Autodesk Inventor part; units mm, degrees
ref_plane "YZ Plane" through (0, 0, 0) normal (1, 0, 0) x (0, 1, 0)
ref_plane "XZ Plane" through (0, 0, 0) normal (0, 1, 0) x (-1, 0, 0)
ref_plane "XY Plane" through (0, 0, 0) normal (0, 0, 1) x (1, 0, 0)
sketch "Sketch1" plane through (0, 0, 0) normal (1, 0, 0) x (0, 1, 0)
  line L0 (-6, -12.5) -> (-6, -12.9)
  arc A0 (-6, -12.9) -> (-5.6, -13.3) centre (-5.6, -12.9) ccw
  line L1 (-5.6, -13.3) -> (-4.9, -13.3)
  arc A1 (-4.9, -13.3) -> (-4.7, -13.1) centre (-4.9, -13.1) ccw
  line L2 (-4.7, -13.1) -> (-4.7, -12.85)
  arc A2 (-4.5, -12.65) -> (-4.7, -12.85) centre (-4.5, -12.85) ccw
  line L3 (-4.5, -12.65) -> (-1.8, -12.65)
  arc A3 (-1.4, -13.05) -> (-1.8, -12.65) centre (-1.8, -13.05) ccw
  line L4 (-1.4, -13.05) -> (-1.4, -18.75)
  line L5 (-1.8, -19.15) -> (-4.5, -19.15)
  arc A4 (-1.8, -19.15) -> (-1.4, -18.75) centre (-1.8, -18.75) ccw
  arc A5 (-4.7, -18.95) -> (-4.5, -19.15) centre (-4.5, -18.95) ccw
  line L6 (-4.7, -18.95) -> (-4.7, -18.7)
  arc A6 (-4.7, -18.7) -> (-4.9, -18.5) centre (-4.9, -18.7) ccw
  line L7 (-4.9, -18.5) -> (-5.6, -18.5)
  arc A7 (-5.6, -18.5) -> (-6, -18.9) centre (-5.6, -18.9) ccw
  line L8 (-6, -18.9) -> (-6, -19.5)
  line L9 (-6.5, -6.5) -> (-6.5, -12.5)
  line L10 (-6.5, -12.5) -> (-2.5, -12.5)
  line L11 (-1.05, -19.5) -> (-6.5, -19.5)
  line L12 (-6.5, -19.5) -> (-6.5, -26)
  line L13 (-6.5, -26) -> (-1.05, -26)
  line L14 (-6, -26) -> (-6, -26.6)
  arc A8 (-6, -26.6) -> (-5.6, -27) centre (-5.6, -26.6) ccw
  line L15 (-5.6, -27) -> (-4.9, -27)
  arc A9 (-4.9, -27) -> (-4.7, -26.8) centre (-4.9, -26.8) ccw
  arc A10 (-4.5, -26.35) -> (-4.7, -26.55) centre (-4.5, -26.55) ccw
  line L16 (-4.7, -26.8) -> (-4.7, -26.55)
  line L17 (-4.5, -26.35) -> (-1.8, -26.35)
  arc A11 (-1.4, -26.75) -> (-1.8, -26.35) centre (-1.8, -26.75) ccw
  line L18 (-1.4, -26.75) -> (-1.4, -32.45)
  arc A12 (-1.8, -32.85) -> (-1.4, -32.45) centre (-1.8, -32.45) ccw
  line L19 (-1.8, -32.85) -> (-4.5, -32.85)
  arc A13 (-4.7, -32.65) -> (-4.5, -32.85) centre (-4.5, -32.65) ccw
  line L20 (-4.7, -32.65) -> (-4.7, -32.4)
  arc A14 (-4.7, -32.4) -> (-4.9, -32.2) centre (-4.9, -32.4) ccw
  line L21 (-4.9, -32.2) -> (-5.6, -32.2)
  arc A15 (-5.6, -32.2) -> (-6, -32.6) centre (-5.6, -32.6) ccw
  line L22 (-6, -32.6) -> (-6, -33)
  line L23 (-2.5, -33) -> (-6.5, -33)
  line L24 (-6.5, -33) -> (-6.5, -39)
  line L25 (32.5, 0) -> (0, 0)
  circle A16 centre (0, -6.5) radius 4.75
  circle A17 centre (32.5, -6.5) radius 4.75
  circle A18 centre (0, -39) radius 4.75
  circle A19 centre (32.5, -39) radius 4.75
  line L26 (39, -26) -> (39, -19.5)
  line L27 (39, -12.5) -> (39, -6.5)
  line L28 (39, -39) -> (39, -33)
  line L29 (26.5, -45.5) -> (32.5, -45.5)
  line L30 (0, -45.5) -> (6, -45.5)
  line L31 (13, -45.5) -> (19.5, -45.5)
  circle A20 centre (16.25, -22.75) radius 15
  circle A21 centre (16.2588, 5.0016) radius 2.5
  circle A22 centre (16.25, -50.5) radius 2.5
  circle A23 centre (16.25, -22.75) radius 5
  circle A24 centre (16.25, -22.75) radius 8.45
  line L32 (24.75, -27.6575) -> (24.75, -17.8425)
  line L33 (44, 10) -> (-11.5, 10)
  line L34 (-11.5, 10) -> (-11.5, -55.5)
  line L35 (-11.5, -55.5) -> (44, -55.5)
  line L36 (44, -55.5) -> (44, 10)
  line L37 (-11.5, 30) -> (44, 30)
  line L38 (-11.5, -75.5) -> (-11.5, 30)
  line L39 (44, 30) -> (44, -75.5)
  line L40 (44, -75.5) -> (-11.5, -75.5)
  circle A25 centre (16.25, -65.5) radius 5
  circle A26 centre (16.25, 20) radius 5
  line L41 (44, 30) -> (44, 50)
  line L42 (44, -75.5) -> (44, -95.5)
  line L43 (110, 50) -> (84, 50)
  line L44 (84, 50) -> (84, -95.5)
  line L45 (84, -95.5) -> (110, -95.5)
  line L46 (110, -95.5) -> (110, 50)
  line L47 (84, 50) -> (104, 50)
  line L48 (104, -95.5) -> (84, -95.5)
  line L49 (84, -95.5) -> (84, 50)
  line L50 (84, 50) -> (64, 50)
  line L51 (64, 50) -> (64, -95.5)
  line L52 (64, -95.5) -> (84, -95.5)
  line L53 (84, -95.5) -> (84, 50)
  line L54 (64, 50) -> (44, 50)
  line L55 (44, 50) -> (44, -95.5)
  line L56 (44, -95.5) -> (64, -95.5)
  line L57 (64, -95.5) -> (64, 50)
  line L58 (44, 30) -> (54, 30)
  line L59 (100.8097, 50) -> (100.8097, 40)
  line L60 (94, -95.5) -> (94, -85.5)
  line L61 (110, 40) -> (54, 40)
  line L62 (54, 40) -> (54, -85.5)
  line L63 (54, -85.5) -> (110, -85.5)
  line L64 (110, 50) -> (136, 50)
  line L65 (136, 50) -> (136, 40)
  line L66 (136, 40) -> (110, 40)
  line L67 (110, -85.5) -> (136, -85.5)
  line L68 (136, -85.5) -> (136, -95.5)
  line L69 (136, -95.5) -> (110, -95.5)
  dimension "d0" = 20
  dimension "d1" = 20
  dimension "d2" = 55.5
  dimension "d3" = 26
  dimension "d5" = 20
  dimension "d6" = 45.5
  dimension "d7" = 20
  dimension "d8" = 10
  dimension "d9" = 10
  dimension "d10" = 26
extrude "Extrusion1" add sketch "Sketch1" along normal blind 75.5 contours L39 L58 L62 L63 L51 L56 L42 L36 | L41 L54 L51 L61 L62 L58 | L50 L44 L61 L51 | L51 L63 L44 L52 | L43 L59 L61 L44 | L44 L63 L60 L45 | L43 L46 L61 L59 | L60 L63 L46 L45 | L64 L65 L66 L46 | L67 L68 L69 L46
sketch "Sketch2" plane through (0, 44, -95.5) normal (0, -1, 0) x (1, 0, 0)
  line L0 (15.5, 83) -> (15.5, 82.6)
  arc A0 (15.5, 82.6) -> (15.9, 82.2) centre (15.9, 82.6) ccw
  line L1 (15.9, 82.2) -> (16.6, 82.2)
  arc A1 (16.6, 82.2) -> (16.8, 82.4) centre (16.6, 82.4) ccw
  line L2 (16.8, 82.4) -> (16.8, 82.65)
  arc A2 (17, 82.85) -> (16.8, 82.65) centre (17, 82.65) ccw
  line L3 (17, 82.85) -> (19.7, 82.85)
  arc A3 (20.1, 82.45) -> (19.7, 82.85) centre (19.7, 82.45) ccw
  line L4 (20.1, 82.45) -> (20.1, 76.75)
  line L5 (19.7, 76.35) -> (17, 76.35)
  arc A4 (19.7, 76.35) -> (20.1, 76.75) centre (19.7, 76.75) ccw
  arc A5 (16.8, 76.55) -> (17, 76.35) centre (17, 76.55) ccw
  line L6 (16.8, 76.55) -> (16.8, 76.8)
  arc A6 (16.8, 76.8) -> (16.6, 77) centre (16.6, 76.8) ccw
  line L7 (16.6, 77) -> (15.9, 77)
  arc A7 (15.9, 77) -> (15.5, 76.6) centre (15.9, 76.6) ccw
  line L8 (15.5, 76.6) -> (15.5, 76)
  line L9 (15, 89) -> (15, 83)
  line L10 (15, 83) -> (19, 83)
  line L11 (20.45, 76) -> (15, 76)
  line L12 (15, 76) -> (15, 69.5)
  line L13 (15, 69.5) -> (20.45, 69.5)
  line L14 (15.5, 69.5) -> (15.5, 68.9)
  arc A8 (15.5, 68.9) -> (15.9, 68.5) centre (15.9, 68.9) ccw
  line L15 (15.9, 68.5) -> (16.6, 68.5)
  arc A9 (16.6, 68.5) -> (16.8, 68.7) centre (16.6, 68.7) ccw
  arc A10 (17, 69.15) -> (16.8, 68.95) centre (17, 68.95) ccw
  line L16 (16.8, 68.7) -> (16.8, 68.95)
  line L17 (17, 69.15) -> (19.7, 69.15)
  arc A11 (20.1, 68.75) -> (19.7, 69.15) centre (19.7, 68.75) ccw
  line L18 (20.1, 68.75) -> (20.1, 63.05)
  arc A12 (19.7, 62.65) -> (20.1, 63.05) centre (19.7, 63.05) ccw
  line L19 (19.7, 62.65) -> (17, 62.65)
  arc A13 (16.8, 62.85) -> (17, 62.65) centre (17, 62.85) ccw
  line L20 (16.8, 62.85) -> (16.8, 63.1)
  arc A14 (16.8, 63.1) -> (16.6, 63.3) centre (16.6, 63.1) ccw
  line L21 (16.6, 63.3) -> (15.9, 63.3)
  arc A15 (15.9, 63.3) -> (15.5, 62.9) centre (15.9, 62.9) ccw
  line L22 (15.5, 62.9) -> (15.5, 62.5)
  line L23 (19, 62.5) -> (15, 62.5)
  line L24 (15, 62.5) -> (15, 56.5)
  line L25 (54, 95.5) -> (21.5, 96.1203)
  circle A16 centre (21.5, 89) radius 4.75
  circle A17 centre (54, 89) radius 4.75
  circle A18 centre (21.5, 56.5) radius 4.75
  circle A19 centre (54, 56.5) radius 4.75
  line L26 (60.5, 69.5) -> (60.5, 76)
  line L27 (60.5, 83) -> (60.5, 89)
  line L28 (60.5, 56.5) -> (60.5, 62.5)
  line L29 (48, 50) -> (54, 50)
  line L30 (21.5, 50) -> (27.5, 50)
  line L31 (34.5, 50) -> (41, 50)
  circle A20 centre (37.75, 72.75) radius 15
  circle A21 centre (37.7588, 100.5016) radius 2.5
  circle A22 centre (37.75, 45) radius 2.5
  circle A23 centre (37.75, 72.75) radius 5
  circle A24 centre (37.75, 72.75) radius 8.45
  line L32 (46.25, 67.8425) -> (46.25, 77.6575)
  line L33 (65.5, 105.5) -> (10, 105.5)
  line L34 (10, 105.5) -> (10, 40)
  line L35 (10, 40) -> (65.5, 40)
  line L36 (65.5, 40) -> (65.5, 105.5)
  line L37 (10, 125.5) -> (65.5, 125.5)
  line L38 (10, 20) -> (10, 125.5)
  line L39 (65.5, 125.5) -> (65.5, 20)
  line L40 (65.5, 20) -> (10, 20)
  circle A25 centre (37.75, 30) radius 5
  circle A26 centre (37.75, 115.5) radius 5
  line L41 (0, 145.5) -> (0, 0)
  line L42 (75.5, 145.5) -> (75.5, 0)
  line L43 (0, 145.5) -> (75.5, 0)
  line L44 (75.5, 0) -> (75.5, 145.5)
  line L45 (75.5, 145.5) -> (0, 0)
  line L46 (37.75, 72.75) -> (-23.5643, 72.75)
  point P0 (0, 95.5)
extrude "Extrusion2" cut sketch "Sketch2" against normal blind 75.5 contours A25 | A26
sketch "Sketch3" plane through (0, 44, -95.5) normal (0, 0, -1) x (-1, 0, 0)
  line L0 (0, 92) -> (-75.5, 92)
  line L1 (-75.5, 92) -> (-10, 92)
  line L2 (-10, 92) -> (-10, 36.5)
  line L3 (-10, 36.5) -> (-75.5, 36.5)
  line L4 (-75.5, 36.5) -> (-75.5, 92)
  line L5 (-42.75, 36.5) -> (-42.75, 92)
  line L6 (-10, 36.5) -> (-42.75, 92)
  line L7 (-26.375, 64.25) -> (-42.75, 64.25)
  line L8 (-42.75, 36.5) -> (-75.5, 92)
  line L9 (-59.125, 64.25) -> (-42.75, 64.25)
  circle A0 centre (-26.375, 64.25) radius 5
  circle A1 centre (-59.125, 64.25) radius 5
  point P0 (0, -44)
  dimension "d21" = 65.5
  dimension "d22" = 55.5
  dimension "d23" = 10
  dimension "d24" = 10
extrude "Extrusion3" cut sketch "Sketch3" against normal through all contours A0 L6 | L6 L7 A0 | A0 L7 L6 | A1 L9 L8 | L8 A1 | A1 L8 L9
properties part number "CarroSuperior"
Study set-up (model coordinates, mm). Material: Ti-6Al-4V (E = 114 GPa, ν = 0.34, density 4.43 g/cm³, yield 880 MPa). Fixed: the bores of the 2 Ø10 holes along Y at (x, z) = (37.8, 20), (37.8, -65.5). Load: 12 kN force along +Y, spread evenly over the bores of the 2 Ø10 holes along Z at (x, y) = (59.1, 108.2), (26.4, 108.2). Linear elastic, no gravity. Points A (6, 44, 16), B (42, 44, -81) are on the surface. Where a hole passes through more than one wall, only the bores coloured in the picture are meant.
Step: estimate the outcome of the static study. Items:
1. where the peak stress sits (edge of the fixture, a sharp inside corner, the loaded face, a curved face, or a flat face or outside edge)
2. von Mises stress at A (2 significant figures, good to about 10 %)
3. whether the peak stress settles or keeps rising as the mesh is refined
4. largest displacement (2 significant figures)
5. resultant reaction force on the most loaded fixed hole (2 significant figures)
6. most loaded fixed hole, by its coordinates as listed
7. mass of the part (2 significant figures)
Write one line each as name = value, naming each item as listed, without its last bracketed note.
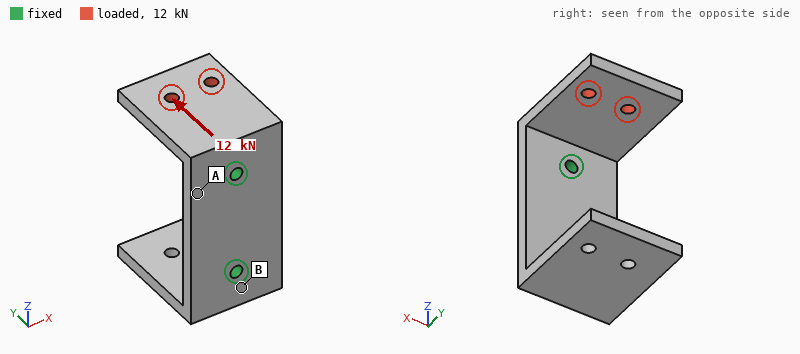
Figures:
where the peak stress sits = edge of the fixture
von Mises stress at A = 63 MPa
whether the peak stress settles or keeps rising as the mesh is refined = keeps rising
largest displacement = 0.60 mm
resultant reaction force on the most loaded fixed hole = 13 kN
most loaded fixed hole, by its coordinates as listed = (37.8, 20)
mass of the part = 1.0 kg
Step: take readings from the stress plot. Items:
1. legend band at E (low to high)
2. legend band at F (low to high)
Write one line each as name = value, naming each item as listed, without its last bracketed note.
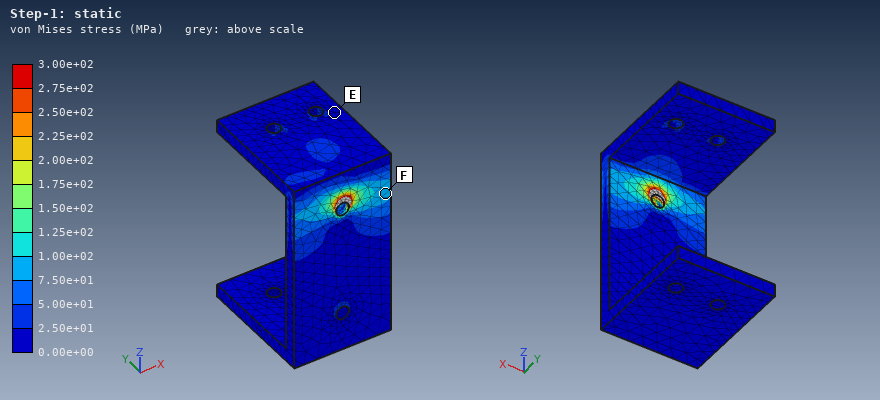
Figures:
legend band at E = 0.00e+00 to 2.50e+01 MPa
legend band at F = 7.50e+01 to 1.00e+02 MPa
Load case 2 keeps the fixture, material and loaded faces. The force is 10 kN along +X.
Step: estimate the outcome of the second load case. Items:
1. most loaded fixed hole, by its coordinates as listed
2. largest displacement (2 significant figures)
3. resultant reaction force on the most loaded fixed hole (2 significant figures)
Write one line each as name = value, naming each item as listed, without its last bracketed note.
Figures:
most loaded fixed hole, by its coordinates as listed = (37.8, 20)
largest displacement = 1.3 mm
resultant reaction force on the most loaded fixed hole = 12 kN
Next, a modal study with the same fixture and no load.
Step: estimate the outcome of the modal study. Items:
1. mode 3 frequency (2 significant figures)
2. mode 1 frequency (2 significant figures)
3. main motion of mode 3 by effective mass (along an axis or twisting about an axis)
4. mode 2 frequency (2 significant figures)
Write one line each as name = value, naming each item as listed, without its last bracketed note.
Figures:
mode 3 frequency = 1100 Hz
mode 1 frequency = 750 Hz
main motion of mode 3 by effective mass = along X
mode 2 frequency = 760 Hz
